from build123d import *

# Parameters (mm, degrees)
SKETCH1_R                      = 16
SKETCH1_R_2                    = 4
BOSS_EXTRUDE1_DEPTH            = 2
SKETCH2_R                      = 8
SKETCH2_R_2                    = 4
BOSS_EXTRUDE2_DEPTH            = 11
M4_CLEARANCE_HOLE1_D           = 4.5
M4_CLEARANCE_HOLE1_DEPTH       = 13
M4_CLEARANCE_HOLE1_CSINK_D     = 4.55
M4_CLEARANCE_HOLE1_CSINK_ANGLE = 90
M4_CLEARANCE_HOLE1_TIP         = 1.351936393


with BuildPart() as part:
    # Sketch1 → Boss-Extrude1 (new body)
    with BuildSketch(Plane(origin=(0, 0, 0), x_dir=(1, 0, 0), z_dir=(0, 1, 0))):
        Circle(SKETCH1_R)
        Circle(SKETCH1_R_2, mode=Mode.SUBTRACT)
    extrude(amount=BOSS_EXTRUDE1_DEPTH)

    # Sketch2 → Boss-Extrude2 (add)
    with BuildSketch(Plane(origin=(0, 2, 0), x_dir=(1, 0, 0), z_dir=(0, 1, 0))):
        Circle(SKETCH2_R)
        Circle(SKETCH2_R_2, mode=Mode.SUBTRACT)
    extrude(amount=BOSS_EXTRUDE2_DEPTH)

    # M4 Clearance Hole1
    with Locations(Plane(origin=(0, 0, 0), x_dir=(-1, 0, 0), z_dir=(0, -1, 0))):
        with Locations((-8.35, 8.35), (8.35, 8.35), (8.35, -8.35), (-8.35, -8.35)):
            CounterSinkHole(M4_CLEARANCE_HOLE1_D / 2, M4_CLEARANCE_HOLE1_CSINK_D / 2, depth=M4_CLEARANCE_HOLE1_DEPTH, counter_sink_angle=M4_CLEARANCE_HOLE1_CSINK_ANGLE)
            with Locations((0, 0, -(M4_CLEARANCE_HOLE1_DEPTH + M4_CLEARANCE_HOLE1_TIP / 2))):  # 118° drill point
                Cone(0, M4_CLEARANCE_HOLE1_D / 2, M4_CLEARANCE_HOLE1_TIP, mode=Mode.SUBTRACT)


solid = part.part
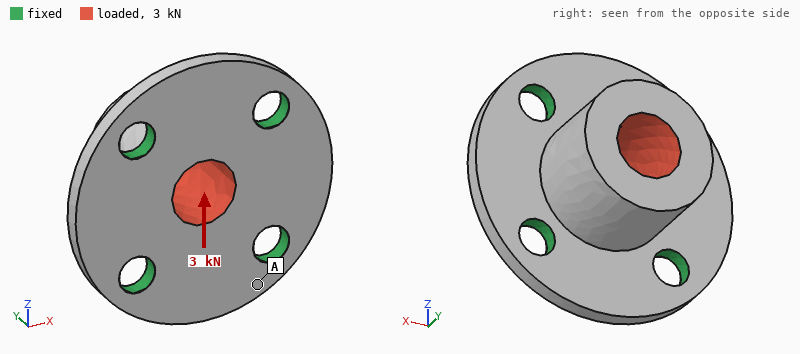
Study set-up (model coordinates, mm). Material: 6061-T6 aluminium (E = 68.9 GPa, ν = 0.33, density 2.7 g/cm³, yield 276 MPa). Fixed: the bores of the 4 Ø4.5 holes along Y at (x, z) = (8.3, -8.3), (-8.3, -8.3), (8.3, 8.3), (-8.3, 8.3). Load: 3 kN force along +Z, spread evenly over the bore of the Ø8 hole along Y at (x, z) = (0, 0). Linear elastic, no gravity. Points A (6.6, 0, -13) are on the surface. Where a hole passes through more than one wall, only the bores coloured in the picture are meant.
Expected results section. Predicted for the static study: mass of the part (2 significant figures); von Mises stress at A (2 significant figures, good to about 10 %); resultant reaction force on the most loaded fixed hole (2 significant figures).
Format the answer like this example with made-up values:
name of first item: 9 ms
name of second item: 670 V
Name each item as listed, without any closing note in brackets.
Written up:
mass of the part: 8.2 g
von Mises stress at A: 22 MPa
resultant reaction force on the most loaded fixed hole: 990 N
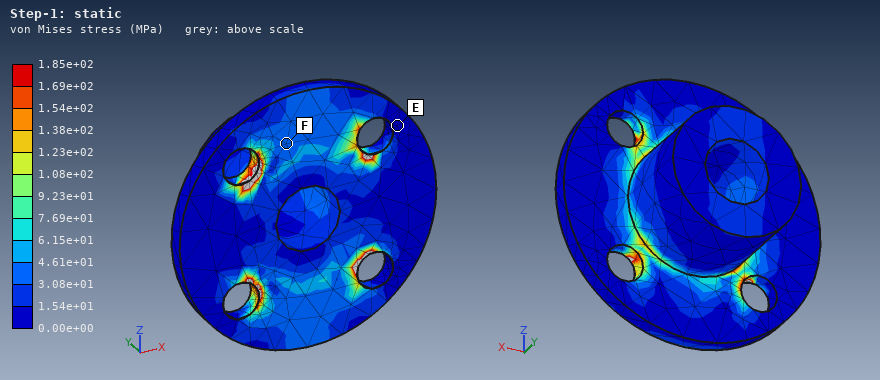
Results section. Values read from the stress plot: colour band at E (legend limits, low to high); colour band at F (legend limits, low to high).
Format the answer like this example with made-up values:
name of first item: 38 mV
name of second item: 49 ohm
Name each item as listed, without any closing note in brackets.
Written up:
colour band at E: 0.00e+00 to 1.54e+01 MPa
colour band at F: 3.08e+01 to 4.61e+01 MPa
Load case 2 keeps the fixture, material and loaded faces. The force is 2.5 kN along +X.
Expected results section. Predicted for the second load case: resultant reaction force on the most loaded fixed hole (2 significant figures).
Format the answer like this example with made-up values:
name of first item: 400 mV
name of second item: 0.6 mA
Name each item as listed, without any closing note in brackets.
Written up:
resultant reaction force on the most loaded fixed hole: 830 N
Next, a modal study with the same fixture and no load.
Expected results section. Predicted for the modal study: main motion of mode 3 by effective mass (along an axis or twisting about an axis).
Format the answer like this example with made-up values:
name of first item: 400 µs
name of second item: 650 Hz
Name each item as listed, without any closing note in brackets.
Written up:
main motion of mode 3 by effective mass: along Y
